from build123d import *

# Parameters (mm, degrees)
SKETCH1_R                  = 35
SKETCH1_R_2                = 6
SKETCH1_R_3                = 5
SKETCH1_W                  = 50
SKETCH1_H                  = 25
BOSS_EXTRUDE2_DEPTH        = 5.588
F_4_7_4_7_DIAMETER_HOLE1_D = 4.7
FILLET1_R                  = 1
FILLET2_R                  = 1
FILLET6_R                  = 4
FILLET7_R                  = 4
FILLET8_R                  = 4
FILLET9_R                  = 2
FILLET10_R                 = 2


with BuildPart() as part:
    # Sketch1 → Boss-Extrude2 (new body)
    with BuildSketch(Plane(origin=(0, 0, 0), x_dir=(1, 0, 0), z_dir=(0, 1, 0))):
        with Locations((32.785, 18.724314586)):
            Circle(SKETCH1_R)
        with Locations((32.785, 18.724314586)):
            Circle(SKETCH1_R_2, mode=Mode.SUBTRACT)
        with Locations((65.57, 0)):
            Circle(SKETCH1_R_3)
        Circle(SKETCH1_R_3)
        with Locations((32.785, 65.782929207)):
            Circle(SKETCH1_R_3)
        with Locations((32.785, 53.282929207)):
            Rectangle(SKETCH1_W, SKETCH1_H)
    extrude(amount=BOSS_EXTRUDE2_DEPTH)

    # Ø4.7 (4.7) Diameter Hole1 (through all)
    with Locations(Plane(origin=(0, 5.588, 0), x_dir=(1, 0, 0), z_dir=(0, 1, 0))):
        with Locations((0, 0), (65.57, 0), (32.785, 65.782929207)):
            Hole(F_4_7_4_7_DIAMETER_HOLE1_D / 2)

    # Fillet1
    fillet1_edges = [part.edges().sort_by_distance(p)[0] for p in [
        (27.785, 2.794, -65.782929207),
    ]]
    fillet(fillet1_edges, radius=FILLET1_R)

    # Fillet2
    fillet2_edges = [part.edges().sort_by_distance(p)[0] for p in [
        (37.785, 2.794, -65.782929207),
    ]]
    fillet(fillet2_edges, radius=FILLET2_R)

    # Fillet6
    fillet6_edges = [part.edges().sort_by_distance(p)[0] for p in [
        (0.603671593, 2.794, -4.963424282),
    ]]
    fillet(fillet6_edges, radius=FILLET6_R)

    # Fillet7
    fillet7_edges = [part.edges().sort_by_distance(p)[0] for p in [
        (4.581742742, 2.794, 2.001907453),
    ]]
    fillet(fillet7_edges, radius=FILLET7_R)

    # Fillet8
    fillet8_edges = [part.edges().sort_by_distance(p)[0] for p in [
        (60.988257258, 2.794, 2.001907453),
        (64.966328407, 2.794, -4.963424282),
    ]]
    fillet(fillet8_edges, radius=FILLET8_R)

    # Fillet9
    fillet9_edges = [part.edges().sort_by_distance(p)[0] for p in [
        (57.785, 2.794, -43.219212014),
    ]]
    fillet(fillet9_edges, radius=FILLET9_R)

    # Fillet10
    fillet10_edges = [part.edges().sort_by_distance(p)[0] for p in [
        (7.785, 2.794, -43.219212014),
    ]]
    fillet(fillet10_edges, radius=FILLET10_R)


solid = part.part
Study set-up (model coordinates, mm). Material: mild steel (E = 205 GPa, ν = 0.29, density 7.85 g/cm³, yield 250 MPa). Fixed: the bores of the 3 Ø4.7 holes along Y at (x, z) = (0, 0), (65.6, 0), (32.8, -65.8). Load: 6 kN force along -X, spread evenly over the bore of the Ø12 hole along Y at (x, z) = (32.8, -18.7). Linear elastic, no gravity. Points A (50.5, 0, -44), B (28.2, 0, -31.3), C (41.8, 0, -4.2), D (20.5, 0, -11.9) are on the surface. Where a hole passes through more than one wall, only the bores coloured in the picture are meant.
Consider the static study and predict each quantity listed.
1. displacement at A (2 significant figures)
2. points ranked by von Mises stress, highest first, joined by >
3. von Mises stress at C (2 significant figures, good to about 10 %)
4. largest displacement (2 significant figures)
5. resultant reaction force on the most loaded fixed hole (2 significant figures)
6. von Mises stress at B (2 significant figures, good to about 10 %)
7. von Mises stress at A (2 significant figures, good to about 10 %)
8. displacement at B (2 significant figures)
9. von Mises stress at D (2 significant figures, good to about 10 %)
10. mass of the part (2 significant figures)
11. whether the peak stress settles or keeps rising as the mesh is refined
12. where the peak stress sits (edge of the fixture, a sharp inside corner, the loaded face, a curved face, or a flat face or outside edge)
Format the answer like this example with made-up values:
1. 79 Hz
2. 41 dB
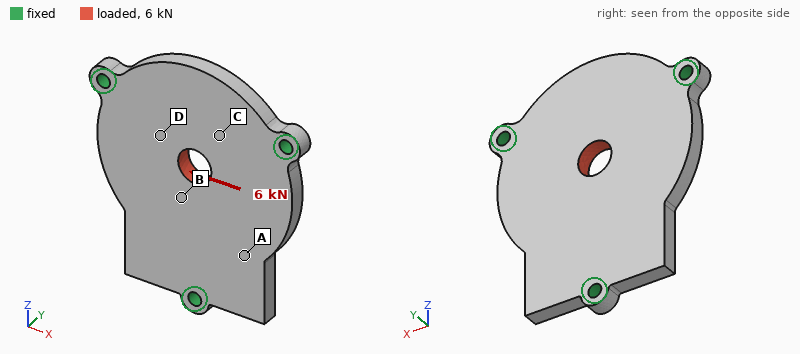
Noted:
1. 3.8 µm
2. D > C > A > B
3. 20 MPa
4. 6.4 µm
5. 2.5 kN
6. 5.6 MPa
7. 9.7 MPa
8. 4.8 µm
9. 27 MPa
10. 200 g
11. keeps rising
12. edge of the fixture
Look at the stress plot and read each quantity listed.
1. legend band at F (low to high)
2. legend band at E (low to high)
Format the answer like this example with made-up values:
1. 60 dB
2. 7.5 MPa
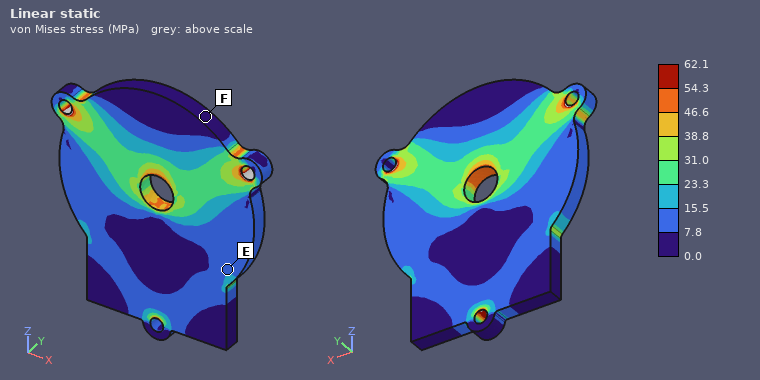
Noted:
1. 0.0 to 7.8 MPa
2. 7.8 to 15.5 MPa
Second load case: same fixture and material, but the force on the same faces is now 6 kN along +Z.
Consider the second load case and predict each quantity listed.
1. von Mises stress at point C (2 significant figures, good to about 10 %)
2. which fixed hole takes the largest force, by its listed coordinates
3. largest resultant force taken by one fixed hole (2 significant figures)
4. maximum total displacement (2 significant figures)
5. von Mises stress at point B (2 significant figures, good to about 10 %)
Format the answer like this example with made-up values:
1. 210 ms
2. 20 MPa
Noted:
1. 14 MPa
2. (32.8, -65.8)
3. 2.5 kN
4. 6.2 µm
5. 27 MPa
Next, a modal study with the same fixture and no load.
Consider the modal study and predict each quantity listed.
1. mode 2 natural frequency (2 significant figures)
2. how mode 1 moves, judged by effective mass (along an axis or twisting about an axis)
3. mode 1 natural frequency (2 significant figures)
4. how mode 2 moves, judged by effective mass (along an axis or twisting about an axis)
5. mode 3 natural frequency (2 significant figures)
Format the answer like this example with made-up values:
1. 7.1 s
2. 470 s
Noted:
1. 4900 Hz
2. along Y
3. 4300 Hz
4. twisting about Z
5. 5500 Hz
